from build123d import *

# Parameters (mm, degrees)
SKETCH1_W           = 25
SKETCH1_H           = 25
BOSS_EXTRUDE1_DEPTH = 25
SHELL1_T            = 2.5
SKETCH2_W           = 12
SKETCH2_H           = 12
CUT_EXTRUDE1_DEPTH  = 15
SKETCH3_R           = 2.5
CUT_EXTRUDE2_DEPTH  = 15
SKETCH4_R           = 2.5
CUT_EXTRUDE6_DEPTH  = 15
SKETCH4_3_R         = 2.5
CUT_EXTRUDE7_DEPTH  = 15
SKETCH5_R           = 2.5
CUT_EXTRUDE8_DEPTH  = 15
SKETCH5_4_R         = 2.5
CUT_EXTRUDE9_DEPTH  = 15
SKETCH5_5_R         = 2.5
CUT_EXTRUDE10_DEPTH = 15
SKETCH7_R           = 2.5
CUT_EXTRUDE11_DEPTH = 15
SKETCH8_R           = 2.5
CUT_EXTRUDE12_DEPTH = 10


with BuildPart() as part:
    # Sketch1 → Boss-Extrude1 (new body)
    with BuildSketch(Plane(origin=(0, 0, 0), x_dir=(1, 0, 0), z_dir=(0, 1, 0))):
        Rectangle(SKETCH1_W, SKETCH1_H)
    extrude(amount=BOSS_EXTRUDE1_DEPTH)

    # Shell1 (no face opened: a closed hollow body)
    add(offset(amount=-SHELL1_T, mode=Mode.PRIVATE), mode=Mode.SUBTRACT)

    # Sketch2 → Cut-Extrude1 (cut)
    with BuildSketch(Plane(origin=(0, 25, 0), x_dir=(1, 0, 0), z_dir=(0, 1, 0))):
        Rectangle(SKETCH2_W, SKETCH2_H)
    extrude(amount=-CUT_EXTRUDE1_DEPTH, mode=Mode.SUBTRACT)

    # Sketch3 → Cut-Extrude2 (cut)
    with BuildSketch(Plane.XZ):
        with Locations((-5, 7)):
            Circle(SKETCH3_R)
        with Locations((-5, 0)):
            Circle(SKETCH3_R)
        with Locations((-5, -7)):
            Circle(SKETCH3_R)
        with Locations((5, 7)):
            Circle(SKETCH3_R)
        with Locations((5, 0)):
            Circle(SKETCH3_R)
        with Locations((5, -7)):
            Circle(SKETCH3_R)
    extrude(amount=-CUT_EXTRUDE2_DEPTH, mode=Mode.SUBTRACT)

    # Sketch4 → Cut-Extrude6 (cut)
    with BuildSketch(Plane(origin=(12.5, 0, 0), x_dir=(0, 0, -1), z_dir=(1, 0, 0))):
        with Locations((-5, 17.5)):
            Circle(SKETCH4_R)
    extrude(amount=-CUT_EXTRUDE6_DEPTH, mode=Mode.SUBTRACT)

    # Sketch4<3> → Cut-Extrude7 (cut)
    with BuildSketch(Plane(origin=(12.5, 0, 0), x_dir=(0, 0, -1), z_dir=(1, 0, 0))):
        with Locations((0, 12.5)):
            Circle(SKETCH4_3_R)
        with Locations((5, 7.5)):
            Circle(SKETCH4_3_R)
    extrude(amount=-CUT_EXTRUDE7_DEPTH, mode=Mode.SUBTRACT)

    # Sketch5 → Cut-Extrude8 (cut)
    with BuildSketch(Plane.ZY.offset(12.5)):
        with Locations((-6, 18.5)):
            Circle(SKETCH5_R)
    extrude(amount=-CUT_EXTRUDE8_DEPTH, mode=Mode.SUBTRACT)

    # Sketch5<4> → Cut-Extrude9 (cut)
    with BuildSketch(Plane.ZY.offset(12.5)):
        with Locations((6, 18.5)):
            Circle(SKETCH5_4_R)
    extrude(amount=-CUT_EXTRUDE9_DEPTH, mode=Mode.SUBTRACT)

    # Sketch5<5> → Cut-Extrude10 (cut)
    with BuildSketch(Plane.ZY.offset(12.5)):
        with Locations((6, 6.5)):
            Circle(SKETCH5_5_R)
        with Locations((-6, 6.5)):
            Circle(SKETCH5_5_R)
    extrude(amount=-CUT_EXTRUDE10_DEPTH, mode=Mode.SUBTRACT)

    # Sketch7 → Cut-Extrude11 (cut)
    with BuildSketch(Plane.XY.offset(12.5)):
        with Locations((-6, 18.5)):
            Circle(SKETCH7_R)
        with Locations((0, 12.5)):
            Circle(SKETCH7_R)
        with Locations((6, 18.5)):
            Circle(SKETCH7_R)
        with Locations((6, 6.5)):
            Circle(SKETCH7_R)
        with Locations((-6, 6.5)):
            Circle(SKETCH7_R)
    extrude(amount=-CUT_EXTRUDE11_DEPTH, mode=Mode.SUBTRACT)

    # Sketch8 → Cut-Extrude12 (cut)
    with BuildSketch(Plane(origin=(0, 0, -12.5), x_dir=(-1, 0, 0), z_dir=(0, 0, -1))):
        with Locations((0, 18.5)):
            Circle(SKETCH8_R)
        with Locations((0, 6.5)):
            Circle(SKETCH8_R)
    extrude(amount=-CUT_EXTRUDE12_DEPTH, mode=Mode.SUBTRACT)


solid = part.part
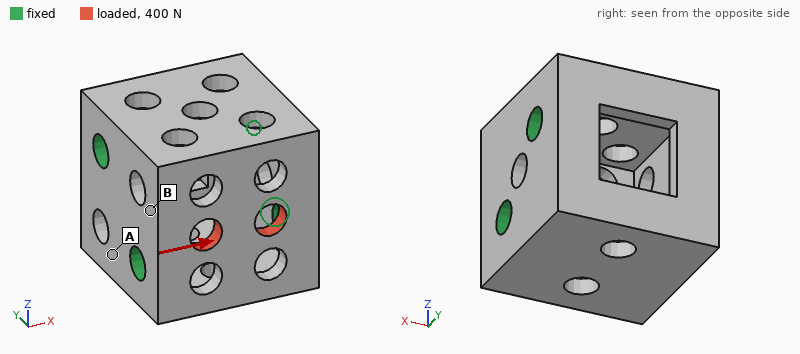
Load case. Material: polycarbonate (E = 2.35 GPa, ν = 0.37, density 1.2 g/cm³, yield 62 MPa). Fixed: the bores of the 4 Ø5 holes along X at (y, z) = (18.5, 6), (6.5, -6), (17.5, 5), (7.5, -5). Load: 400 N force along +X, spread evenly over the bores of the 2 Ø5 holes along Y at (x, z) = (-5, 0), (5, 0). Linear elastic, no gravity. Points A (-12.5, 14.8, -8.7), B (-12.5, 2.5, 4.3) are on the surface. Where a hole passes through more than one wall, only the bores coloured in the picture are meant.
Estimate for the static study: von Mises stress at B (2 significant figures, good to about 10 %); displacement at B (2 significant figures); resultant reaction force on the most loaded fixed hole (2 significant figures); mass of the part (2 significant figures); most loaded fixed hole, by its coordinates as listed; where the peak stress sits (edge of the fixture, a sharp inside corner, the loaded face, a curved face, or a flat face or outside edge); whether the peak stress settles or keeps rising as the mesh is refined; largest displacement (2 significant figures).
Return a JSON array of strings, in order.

["7.8 MPa", "0.088 mm", "180 N", "7.5 g", "(6.5, -6)", "edge of the fixture", "keeps rising", "0.13 mm"]
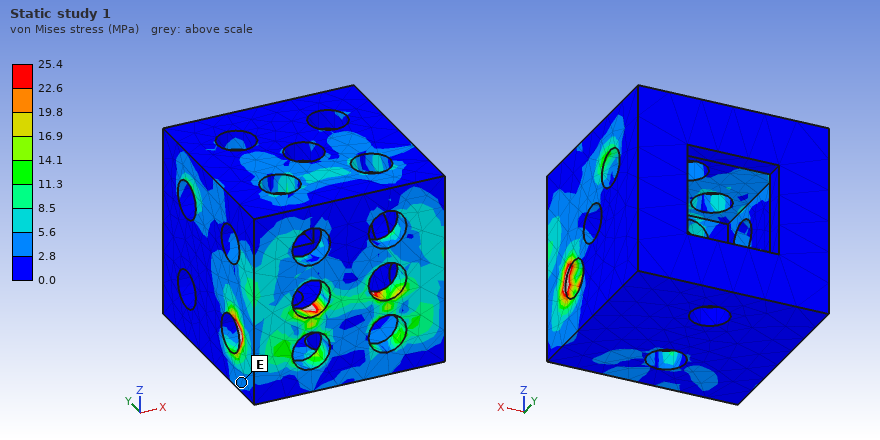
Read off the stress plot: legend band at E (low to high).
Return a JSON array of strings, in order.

["2.8 to 5.6 MPa"]
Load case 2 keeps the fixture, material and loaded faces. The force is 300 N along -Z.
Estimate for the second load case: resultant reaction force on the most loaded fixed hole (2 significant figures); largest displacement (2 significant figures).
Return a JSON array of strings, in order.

["160 N", "78 µm"]
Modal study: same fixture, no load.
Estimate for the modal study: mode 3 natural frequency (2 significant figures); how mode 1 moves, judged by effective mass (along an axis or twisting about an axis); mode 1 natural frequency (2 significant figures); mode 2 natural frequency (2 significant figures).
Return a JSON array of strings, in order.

["7200 Hz", "along X", "6300 Hz", "7000 Hz"]
